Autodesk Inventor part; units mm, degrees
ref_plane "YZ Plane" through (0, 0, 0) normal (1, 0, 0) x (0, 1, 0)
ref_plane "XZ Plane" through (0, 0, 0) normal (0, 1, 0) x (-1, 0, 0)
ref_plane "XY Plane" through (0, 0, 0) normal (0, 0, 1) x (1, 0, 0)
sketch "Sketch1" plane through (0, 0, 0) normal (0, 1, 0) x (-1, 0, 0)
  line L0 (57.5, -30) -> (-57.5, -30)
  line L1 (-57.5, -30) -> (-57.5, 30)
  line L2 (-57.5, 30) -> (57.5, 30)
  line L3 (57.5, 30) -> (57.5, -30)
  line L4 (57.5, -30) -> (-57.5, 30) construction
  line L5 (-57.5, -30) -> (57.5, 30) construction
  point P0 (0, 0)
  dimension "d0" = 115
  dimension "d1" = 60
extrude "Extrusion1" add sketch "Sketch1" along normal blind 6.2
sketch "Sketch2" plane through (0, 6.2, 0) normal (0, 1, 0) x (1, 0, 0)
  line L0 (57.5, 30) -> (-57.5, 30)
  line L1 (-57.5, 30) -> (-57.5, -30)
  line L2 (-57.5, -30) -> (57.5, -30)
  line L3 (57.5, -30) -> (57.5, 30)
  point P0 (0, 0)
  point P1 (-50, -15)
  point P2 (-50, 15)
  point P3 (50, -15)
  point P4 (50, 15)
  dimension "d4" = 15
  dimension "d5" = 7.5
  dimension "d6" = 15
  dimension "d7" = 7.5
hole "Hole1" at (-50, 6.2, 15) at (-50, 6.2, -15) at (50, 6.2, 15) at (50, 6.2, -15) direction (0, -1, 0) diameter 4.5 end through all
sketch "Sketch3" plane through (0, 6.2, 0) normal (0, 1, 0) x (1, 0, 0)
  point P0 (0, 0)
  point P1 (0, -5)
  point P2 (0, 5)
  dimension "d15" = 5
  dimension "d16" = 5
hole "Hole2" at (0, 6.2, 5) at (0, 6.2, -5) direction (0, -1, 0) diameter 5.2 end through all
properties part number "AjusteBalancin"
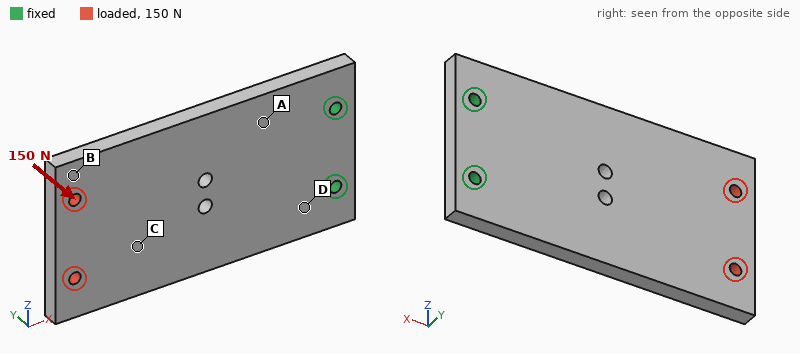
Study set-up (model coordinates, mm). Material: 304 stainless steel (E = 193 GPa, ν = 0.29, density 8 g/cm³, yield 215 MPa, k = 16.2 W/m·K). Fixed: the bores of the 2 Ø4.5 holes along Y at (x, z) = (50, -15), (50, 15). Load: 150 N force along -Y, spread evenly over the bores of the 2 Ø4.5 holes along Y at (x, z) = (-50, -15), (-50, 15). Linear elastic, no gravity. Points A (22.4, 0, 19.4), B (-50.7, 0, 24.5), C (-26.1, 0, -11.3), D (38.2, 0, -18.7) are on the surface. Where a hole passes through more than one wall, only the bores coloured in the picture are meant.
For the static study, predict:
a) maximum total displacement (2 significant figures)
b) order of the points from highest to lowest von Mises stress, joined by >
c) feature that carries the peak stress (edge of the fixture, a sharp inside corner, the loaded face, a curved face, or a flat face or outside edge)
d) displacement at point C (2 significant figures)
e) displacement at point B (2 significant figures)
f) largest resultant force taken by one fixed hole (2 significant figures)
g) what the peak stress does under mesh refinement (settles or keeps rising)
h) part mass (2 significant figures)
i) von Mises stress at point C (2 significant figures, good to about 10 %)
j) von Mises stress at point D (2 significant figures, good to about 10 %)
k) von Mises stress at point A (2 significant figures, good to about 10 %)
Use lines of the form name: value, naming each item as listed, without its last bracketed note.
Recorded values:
maximum total displacement: 0.26 mm
order of the points from highest to lowest von Mises stress, joined by >: D > A > C > B
feature that carries the peak stress: edge of the fixture
displacement at point C: 0.15 mm
displacement at point B: 0.23 mm
largest resultant force taken by one fixed hole: 75 N
what the peak stress does under mesh refinement: keeps rising
part mass: 340 g
von Mises stress at point C: 9.7 MPa
von Mises stress at point D: 33 MPa
von Mises stress at point A: 27 MPa
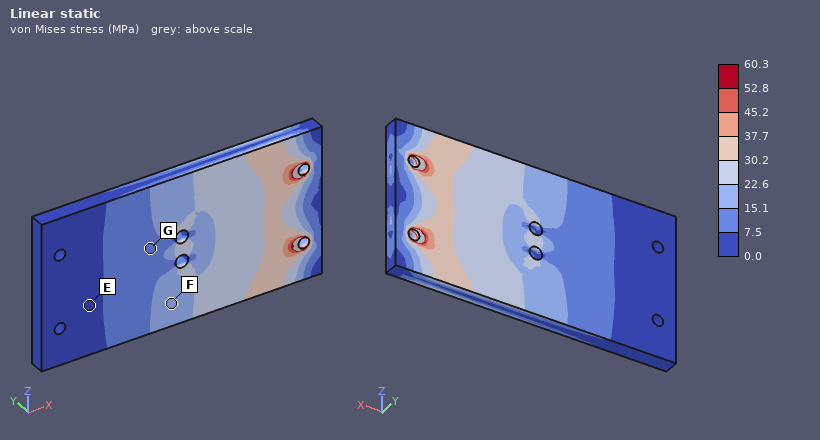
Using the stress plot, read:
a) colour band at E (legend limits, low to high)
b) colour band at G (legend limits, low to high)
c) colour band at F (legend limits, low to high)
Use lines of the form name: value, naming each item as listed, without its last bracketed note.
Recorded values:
colour band at E: 0.0 to 7.5 MPa
colour band at G: 7.5 to 15.1 MPa
colour band at F: 15.1 to 22.6 MPa
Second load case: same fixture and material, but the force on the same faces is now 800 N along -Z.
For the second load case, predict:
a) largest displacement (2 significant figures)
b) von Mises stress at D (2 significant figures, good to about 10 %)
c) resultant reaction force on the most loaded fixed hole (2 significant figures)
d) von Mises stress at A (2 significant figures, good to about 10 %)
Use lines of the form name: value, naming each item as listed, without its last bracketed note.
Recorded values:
largest displacement: 27 µm
von Mises stress at D: 17 MPa
resultant reaction force on the most loaded fixed hole: 2.5 kN
von Mises stress at A: 11 MPa
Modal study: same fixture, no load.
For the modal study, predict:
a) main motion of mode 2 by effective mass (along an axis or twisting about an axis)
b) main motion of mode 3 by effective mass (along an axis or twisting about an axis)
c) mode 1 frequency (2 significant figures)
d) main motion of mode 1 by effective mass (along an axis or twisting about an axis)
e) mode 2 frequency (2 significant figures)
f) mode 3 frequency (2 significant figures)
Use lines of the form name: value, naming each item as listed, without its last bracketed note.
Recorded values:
main motion of mode 2 by effective mass: twisting about X
main motion of mode 3 by effective mass: along Y
mode 1 frequency: 420 Hz
main motion of mode 1 by effective mass: along Y
mode 2 frequency: 1600 Hz
mode 3 frequency: 2500 Hz
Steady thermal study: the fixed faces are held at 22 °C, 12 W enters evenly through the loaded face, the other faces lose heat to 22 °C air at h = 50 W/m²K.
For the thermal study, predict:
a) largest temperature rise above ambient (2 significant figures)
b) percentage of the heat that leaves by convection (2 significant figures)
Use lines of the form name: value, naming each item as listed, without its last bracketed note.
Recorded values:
largest temperature rise above ambient: 57 K
percentage of the heat that leaves by convection: 95 %
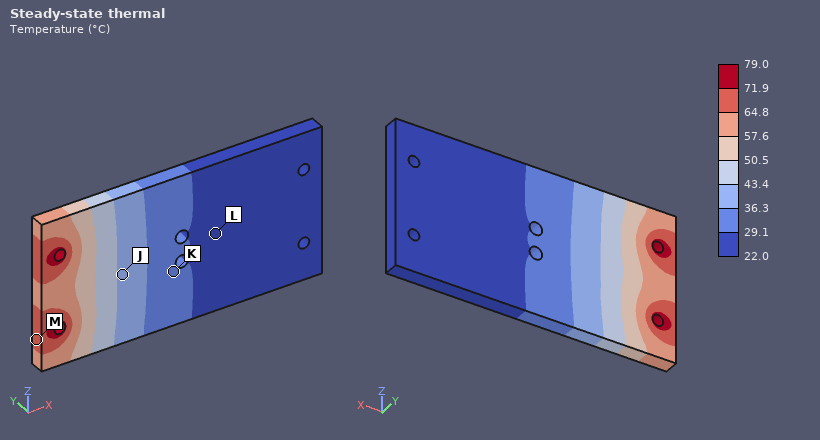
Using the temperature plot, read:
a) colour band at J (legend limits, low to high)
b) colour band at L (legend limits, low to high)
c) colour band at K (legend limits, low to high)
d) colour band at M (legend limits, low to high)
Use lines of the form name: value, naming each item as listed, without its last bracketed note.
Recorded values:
colour band at J: 36.3 to 43.4 °C
colour band at L: 22.0 to 29.1 °C
colour band at K: 29.1 to 36.3 °C
colour band at M: 64.8 to 71.9 °C
